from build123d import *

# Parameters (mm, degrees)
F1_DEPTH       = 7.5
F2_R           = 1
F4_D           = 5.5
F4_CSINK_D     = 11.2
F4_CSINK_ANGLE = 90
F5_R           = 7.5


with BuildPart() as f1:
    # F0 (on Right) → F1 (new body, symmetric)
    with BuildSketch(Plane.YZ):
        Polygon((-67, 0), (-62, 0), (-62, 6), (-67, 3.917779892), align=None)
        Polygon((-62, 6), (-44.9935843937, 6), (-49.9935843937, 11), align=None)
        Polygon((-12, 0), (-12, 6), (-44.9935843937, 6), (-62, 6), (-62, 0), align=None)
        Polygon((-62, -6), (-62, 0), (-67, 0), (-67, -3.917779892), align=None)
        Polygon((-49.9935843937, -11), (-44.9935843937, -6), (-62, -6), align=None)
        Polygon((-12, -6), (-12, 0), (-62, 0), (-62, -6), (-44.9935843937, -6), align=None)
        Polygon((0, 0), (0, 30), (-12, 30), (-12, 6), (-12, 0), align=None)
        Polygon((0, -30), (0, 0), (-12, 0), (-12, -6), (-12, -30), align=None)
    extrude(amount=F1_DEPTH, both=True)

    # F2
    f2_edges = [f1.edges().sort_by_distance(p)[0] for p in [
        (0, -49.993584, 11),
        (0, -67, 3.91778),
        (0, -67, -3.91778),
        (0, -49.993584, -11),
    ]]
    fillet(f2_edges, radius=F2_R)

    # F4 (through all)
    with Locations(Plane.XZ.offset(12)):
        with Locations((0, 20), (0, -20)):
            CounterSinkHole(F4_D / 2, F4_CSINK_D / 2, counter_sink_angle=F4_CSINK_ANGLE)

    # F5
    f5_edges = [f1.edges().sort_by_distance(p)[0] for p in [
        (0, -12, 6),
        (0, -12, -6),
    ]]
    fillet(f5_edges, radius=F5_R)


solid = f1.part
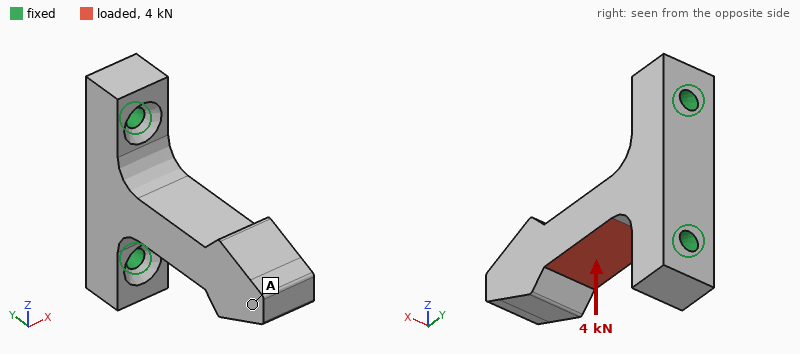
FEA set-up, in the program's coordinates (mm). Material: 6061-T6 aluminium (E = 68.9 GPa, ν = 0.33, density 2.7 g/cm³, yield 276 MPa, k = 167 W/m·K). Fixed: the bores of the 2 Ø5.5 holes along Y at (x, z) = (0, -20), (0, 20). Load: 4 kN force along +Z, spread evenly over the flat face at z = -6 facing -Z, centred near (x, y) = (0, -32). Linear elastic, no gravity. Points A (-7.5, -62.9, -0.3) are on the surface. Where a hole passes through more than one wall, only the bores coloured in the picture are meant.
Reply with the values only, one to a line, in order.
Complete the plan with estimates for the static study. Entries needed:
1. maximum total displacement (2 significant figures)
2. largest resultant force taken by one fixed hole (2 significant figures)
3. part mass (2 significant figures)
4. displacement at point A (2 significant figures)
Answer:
0.33 mm
3.8 kN
58 g
0.30 mm
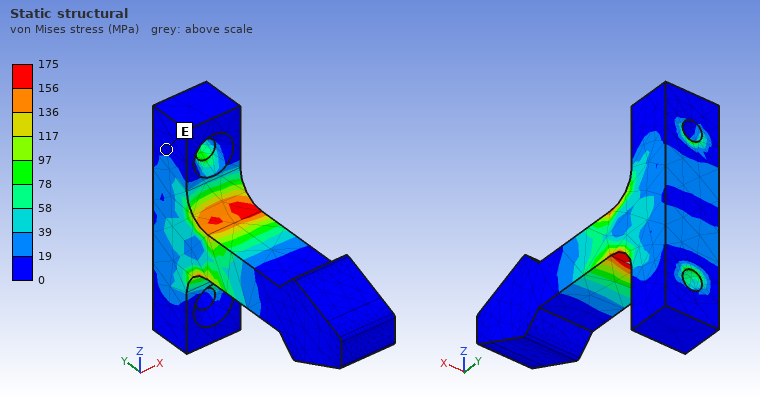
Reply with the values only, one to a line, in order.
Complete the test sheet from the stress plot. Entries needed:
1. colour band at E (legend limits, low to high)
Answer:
0 to 19 MPa
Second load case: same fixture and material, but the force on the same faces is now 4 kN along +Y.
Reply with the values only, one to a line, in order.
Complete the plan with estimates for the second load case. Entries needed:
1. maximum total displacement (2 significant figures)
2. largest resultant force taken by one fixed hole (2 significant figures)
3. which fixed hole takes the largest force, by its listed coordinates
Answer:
0.15 mm
2.9 kN
(0, -20)
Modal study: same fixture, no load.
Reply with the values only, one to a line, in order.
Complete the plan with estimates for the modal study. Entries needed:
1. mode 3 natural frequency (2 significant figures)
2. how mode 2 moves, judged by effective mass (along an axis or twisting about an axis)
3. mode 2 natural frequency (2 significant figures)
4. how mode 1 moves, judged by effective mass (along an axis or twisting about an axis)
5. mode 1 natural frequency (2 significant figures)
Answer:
11 kHz
along Z
2900 Hz
along X
2300 Hz
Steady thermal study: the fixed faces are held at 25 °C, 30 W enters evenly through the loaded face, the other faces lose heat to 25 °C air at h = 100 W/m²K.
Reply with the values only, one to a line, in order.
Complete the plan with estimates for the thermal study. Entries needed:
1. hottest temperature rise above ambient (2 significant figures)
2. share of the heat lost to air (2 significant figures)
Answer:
23 K
20 %
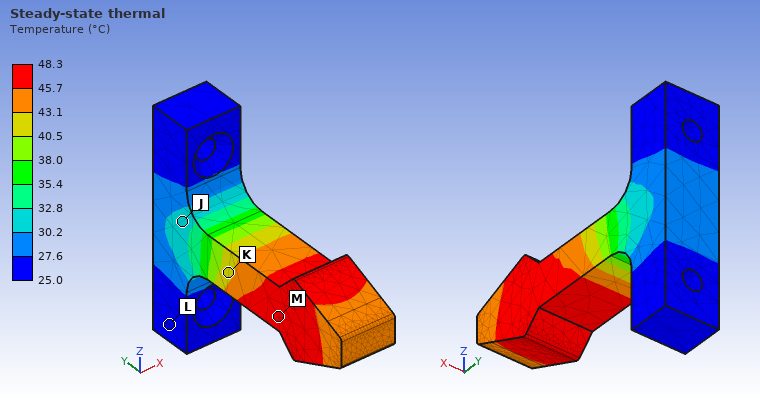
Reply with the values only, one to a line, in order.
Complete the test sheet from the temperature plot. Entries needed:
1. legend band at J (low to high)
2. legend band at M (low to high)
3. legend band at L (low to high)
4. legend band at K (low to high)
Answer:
30.2 to 32.8 °C
45.7 to 48.3 °C
25.0 to 27.6 °C
40.5 to 43.1 °C
